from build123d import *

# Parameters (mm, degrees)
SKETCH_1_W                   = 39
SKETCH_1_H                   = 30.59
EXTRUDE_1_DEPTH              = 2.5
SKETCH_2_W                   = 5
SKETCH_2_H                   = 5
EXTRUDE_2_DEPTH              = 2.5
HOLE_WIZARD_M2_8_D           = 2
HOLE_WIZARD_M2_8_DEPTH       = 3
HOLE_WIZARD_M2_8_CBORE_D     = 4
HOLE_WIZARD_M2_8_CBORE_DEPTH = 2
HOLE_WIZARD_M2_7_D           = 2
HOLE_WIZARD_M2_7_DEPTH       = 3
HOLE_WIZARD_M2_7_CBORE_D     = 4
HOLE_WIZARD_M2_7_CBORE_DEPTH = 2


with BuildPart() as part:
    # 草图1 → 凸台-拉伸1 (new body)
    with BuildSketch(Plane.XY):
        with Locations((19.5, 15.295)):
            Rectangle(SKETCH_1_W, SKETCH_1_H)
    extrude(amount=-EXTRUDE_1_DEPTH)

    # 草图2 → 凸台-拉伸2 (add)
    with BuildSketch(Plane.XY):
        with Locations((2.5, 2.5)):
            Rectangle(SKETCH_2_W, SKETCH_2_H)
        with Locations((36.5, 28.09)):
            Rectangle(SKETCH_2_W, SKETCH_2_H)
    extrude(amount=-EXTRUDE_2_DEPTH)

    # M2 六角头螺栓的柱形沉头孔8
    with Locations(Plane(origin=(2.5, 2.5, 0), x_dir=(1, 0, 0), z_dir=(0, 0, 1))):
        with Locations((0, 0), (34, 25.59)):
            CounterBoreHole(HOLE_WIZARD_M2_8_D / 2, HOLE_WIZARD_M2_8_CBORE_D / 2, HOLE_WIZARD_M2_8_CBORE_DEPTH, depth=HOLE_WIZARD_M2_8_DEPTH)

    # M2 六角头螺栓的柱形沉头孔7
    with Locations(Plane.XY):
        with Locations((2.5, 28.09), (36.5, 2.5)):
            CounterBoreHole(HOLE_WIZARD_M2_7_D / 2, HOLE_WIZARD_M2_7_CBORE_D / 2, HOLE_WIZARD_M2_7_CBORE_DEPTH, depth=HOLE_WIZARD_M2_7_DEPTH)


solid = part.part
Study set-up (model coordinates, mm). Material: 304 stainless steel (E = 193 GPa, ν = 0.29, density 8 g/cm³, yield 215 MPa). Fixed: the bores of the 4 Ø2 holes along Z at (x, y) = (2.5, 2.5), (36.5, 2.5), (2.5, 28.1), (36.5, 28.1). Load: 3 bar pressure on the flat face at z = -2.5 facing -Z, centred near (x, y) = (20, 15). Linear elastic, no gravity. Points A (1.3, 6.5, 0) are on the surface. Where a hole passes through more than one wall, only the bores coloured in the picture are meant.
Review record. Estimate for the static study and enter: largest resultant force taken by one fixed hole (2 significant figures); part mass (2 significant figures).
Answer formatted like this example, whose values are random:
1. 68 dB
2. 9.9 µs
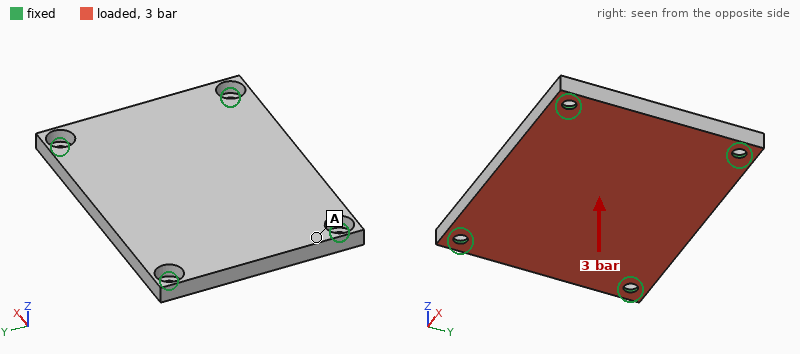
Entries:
1. 190 N
2. 23 g
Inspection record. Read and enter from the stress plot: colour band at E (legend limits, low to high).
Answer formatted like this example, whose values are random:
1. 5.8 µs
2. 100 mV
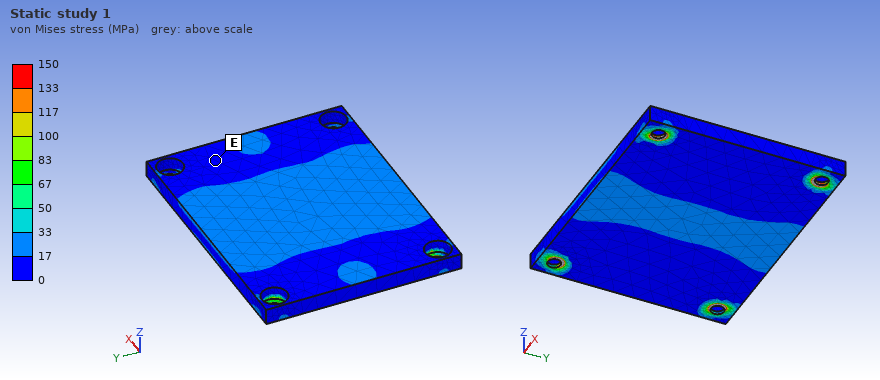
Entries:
1. 0 to 17 MPa
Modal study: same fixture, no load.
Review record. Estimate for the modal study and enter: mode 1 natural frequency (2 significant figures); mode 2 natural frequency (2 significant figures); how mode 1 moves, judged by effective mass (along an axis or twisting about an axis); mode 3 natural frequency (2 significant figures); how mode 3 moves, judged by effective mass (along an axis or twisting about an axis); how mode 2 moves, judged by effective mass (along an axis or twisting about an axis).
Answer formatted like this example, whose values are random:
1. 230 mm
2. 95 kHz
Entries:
1. 6000 Hz
2. 10000 Hz
3. along Z
4. 13 kHz
5. twisting about Y
6. twisting about X
